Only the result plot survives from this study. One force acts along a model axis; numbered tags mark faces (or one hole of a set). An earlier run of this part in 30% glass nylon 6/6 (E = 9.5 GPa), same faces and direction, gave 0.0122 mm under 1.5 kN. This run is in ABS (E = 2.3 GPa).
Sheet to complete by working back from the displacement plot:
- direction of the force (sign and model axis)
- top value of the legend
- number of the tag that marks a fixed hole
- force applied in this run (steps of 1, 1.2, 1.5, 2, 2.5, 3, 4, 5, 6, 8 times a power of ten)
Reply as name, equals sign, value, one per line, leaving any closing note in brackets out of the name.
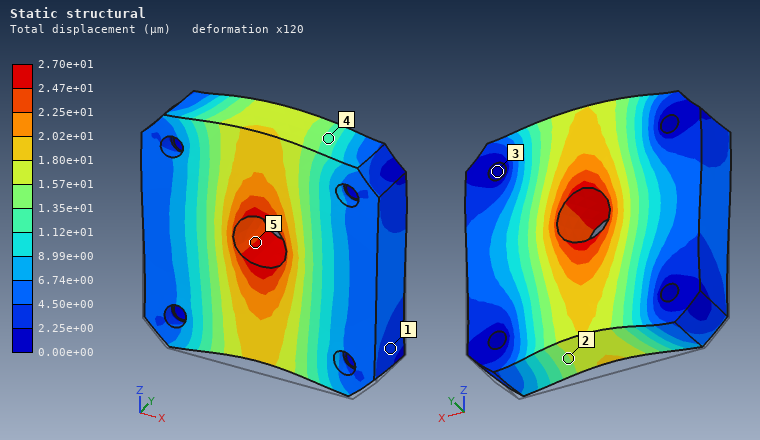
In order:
direction of the force = +Z
top value of the legend = 2.70e+01 µm
number of the tag that marks a fixed hole = 3
force applied in this run = 800 N
